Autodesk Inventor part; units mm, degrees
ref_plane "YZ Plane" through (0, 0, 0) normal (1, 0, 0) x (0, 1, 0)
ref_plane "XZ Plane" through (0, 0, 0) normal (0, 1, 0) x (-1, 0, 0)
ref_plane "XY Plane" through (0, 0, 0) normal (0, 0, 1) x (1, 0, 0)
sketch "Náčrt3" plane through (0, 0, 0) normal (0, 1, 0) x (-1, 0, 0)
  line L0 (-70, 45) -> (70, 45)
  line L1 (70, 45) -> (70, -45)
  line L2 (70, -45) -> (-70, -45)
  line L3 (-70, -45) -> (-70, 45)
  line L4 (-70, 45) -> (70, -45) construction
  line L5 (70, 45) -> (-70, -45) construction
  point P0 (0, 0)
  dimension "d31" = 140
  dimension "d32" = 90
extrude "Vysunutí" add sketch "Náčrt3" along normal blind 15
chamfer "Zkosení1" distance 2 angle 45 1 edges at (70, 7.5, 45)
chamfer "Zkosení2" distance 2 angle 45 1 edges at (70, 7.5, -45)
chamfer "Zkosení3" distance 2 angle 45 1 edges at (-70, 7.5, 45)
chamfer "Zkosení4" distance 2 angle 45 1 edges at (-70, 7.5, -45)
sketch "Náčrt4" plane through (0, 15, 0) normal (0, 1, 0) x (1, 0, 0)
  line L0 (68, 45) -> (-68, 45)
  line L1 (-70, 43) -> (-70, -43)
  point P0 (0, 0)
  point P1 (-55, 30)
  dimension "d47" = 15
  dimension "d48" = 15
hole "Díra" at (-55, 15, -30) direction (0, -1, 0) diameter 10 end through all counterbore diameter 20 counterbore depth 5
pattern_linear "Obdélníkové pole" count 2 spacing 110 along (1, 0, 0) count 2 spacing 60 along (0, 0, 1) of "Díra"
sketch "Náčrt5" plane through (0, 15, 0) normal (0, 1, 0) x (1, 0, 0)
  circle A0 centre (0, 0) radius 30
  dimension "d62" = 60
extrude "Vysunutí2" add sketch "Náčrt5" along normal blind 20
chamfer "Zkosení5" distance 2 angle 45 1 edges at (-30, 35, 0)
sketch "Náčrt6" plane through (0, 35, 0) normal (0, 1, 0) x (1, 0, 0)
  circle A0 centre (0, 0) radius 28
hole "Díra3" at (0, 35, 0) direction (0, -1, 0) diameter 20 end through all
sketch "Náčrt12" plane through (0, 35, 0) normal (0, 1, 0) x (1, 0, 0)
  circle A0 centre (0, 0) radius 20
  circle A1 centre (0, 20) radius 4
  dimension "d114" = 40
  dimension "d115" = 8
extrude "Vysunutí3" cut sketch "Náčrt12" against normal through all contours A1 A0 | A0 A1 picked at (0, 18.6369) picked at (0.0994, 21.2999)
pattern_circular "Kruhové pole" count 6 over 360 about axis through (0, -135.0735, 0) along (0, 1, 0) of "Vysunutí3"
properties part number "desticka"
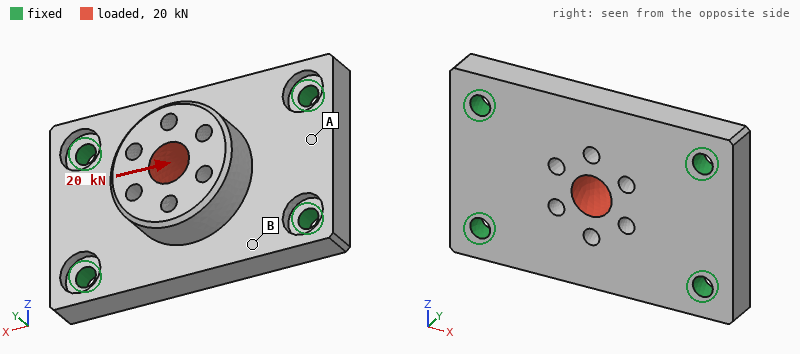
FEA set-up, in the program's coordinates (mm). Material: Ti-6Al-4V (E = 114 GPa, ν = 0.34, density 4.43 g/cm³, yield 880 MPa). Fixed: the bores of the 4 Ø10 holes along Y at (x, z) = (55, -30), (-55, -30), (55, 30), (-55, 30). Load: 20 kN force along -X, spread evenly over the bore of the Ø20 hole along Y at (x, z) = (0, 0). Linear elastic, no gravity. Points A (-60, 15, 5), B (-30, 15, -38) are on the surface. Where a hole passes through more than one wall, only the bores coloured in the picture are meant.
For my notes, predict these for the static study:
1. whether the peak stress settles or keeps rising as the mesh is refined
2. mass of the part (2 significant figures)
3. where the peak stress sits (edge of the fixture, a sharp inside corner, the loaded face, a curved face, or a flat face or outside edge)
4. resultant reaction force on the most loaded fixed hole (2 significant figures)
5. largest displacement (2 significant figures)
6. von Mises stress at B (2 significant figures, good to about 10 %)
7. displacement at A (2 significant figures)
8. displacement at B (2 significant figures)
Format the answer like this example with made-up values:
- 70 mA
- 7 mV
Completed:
- keeps rising
- 950 g
- edge of the fixture
- 5.4 kN
- 12 µm
- 8.2 MPa
- 2.8 µm
- 2.2 µm
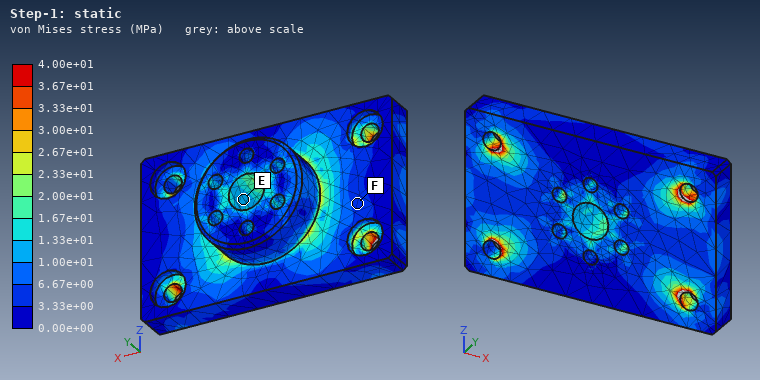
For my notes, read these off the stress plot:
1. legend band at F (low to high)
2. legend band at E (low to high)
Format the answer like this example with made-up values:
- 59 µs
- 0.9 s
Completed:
- 3.33e+00 to 6.67e+00 MPa
- 1.00e+01 to 1.33e+01 MPa
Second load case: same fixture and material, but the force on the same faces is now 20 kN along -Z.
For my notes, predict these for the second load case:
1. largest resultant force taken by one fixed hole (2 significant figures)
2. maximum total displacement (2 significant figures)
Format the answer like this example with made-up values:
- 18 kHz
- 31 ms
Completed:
- 6.7 kN
- 26 µm
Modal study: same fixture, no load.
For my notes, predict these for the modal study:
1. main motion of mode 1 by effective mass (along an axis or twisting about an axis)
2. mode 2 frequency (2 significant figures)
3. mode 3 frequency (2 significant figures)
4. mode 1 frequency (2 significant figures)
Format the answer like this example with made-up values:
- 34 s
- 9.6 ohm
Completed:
- along Y
- 5700 Hz
- 9900 Hz
- 4800 Hz
